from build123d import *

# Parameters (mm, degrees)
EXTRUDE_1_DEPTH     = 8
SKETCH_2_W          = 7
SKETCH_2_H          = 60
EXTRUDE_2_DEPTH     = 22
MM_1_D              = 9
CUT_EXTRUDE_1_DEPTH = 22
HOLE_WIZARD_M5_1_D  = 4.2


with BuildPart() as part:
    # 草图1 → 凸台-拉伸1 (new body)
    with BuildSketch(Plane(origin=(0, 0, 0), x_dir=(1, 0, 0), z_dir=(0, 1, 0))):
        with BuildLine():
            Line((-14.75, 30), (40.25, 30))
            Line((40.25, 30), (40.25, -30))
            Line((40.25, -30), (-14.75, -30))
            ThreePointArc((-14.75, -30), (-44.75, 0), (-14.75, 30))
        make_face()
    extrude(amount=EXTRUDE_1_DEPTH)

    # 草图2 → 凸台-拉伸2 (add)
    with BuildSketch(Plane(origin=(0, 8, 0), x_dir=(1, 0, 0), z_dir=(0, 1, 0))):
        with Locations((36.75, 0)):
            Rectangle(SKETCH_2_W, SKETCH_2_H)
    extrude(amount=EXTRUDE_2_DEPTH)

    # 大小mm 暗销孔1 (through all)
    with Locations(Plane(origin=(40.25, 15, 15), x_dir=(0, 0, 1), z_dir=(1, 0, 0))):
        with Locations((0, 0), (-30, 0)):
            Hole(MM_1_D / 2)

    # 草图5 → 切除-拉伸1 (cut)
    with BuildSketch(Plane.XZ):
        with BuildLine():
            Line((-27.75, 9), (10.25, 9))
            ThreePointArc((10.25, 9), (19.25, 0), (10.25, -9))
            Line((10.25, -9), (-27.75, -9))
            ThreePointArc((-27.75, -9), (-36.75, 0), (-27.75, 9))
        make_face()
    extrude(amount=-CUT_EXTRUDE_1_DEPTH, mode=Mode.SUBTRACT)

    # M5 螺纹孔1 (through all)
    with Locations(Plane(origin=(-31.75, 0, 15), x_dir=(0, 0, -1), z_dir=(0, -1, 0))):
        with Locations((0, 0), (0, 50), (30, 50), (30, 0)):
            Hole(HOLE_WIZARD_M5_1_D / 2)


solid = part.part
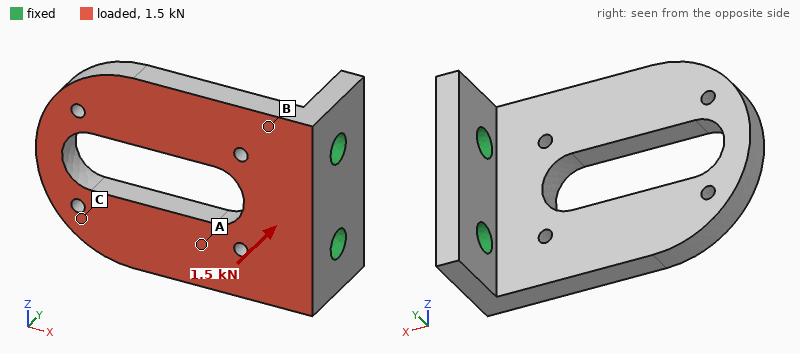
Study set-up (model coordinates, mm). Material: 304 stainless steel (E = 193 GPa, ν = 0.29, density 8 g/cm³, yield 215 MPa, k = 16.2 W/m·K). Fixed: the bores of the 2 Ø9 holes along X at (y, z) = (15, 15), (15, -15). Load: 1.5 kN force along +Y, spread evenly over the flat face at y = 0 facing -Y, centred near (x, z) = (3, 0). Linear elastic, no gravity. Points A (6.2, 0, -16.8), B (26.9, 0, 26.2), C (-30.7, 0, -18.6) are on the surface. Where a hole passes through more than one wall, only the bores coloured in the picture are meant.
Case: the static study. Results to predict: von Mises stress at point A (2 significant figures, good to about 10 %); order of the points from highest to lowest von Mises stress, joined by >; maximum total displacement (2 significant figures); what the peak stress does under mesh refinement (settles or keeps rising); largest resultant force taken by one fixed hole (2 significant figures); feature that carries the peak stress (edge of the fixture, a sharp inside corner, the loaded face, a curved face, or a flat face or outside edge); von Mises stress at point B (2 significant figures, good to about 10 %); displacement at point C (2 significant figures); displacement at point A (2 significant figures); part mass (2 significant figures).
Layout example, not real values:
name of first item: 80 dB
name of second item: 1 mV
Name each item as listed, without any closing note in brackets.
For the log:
von Mises stress at point A: 40 MPa
order of the points from highest to lowest von Mises stress, joined by >: B > A > C
maximum total displacement: 0.28 mm
what the peak stress does under mesh refinement: keeps rising
largest resultant force taken by one fixed hole: 760 N
feature that carries the peak stress: edge of the fixture
von Mises stress at point B: 67 MPa
displacement at point C: 0.22 mm
displacement at point A: 0.074 mm
part mass: 300 g
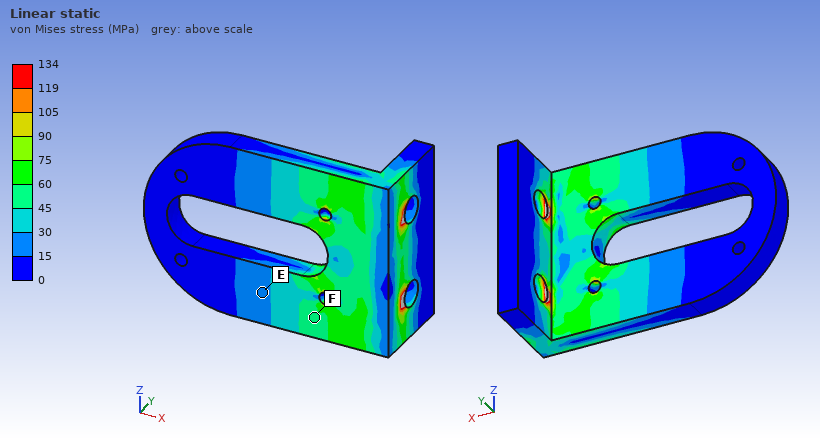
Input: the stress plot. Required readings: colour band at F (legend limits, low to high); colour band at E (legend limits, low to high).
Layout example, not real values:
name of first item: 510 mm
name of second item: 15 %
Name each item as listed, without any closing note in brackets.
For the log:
colour band at F: 45 to 60 MPa
colour band at E: 15 to 30 MPa
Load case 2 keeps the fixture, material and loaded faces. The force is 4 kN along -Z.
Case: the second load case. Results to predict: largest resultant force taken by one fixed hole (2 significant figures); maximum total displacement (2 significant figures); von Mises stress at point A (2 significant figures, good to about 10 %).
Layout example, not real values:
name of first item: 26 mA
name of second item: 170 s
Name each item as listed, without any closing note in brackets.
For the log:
largest resultant force taken by one fixed hole: 4.3 kN
maximum total displacement: 61 µm
von Mises stress at point A: 33 MPa
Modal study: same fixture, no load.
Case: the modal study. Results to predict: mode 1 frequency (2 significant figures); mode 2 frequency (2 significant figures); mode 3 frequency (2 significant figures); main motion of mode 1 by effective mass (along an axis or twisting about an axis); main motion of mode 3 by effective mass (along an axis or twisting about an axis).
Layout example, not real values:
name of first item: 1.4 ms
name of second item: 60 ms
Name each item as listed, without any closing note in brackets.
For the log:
mode 1 frequency: 970 Hz
mode 2 frequency: 2600 Hz
mode 3 frequency: 3300 Hz
main motion of mode 1 by effective mass: along Y
main motion of mode 3 by effective mass: along Z
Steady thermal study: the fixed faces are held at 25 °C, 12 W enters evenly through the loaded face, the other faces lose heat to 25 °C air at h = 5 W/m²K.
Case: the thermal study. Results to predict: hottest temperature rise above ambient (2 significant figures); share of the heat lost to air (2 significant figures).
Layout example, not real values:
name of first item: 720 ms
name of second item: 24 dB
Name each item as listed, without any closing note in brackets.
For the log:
hottest temperature rise above ambient: 68 K
share of the heat lost to air: 14 %
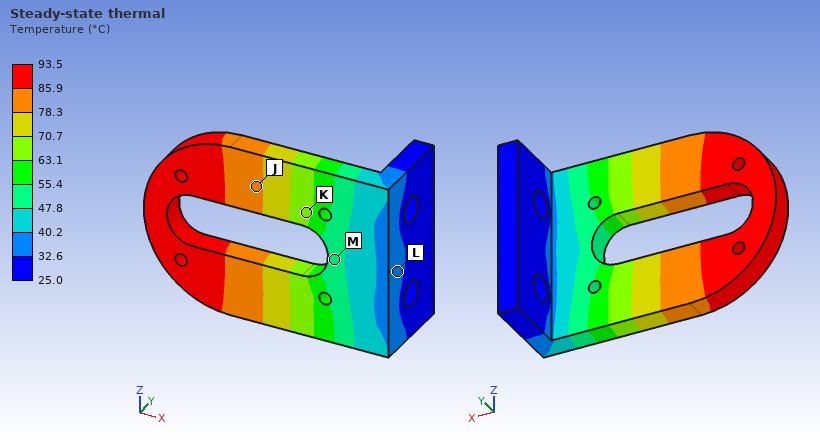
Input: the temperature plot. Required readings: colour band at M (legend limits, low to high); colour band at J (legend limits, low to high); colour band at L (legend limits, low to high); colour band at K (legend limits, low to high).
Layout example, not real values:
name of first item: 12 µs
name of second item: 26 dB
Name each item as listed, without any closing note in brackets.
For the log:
colour band at M: 47.8 to 55.4 °C
colour band at J: 78.3 to 85.9 °C
colour band at L: 32.6 to 40.2 °C
colour band at K: 63.1 to 70.7 °C
